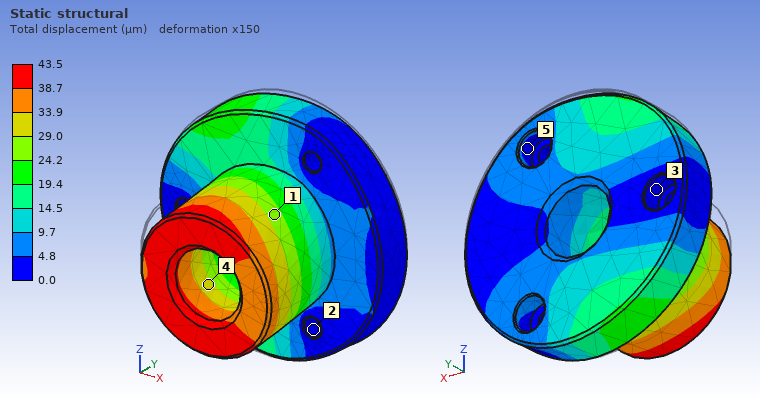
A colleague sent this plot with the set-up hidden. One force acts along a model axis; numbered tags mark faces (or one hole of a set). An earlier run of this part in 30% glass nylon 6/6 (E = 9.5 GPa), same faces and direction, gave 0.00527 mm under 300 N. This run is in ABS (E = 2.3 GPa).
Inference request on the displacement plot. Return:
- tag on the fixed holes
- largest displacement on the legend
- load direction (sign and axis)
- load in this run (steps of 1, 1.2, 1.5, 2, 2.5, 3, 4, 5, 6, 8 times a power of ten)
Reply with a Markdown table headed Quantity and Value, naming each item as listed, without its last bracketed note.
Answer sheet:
| Quantity | Value |
|---|---|
| tag on the fixed holes | 2 |
| largest displacement on the legend | 43.5 µm |
| load direction | -Z |
| load in this run | 600 N |
